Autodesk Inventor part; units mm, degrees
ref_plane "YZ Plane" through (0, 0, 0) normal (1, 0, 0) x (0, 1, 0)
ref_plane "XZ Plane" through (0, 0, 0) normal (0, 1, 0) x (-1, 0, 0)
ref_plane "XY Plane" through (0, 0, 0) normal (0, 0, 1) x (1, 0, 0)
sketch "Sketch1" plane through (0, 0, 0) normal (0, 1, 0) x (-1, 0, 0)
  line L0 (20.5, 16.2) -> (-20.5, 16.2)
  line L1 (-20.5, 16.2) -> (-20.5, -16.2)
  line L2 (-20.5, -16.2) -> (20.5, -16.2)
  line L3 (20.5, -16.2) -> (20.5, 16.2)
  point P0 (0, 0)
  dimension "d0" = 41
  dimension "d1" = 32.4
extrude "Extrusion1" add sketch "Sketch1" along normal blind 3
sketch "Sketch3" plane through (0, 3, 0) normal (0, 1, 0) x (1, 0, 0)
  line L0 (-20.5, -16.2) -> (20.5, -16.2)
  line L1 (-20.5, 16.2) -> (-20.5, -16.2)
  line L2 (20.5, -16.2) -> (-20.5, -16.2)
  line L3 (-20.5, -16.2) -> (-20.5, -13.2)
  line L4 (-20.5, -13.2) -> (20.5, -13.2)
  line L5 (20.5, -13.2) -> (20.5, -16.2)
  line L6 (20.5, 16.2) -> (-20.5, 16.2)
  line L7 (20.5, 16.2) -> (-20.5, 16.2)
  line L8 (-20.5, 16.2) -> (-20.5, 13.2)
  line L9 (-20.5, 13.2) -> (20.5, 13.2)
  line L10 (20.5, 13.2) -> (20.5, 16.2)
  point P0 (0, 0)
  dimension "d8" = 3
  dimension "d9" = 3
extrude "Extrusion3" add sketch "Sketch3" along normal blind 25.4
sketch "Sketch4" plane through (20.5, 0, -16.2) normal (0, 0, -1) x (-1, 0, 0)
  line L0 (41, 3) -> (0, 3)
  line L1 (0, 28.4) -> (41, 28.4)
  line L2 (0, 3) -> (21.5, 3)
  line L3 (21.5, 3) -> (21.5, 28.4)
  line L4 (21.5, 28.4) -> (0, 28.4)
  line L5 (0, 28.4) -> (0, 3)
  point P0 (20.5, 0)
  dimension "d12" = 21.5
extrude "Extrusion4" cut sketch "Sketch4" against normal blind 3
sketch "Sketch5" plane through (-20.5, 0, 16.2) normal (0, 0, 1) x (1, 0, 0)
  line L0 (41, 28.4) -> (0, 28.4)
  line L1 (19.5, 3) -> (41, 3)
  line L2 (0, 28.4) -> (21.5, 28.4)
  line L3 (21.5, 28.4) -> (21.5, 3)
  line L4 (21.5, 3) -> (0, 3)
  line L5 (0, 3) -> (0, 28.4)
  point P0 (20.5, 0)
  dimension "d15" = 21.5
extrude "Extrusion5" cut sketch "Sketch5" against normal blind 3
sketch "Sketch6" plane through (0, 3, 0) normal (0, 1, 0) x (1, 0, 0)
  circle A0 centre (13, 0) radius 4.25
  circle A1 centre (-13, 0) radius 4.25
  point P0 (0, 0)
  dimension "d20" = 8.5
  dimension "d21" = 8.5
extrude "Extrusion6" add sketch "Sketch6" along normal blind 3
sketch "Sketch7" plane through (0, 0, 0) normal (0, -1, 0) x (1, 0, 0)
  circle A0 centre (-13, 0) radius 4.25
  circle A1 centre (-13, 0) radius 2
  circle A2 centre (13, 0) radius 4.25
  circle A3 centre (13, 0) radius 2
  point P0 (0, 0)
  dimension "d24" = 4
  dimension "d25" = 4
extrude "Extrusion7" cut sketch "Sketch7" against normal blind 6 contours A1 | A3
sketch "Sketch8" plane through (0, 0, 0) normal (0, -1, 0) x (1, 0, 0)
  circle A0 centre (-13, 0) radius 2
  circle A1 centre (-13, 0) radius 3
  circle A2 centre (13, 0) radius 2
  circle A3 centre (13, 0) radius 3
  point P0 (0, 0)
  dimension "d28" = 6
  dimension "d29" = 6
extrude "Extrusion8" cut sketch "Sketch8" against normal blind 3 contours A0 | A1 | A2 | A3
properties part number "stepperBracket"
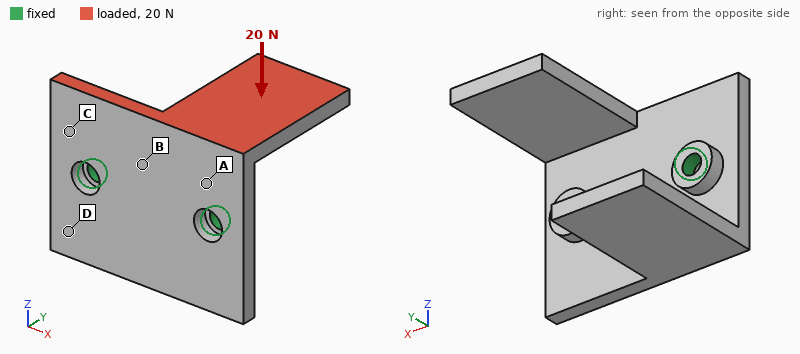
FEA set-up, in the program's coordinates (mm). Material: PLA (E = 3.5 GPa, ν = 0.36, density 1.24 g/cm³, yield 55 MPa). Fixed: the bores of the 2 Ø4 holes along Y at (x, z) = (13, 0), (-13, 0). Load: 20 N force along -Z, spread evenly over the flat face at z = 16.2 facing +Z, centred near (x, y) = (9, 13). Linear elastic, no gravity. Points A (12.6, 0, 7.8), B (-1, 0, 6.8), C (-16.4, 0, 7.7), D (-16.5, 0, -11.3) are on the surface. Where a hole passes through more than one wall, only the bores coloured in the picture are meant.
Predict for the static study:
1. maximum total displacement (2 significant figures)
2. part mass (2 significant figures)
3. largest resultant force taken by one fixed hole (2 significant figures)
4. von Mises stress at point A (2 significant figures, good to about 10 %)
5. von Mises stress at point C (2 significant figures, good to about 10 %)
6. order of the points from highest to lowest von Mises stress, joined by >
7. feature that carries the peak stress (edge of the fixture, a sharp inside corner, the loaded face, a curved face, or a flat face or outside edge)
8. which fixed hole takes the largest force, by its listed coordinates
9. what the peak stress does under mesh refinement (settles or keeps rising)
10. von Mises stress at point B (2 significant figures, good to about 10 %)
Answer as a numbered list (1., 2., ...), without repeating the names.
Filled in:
1. 0.64 mm
2. 8.7 g
3. 17 N
4. 4.7 MPa
5. 1.9 MPa
6. A > B > C > D
7. a sharp inside corner
8. (13, 0)
9. keeps rising
10. 3.2 MPa
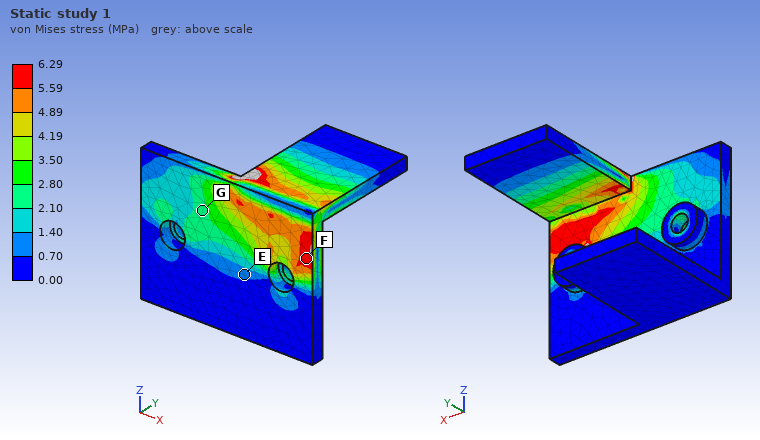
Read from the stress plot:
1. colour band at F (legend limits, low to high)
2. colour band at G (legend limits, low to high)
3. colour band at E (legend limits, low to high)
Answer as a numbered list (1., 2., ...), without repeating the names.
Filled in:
1. 5.59 to 6.29 MPa
2. 2.10 to 2.80 MPa
3. 0.70 to 1.40 MPa
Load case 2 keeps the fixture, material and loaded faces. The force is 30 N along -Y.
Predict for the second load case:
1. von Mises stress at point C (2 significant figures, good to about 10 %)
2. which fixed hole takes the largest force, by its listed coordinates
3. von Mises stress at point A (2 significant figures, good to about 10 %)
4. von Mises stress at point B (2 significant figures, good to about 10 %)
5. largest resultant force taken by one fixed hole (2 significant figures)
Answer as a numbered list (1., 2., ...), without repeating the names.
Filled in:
1. 3.4 MPa
2. (13, 0)
3. 5.0 MPa
4. 4.2 MPa
5. 25 N
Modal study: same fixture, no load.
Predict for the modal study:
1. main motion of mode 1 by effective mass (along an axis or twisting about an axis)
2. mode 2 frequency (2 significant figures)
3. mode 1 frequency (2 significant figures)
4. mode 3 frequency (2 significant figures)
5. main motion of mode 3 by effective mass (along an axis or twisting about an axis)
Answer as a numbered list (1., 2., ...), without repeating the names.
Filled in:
1. along Z
2. 710 Hz
3. 670 Hz
4. 1200 Hz
5. twisting about Y
